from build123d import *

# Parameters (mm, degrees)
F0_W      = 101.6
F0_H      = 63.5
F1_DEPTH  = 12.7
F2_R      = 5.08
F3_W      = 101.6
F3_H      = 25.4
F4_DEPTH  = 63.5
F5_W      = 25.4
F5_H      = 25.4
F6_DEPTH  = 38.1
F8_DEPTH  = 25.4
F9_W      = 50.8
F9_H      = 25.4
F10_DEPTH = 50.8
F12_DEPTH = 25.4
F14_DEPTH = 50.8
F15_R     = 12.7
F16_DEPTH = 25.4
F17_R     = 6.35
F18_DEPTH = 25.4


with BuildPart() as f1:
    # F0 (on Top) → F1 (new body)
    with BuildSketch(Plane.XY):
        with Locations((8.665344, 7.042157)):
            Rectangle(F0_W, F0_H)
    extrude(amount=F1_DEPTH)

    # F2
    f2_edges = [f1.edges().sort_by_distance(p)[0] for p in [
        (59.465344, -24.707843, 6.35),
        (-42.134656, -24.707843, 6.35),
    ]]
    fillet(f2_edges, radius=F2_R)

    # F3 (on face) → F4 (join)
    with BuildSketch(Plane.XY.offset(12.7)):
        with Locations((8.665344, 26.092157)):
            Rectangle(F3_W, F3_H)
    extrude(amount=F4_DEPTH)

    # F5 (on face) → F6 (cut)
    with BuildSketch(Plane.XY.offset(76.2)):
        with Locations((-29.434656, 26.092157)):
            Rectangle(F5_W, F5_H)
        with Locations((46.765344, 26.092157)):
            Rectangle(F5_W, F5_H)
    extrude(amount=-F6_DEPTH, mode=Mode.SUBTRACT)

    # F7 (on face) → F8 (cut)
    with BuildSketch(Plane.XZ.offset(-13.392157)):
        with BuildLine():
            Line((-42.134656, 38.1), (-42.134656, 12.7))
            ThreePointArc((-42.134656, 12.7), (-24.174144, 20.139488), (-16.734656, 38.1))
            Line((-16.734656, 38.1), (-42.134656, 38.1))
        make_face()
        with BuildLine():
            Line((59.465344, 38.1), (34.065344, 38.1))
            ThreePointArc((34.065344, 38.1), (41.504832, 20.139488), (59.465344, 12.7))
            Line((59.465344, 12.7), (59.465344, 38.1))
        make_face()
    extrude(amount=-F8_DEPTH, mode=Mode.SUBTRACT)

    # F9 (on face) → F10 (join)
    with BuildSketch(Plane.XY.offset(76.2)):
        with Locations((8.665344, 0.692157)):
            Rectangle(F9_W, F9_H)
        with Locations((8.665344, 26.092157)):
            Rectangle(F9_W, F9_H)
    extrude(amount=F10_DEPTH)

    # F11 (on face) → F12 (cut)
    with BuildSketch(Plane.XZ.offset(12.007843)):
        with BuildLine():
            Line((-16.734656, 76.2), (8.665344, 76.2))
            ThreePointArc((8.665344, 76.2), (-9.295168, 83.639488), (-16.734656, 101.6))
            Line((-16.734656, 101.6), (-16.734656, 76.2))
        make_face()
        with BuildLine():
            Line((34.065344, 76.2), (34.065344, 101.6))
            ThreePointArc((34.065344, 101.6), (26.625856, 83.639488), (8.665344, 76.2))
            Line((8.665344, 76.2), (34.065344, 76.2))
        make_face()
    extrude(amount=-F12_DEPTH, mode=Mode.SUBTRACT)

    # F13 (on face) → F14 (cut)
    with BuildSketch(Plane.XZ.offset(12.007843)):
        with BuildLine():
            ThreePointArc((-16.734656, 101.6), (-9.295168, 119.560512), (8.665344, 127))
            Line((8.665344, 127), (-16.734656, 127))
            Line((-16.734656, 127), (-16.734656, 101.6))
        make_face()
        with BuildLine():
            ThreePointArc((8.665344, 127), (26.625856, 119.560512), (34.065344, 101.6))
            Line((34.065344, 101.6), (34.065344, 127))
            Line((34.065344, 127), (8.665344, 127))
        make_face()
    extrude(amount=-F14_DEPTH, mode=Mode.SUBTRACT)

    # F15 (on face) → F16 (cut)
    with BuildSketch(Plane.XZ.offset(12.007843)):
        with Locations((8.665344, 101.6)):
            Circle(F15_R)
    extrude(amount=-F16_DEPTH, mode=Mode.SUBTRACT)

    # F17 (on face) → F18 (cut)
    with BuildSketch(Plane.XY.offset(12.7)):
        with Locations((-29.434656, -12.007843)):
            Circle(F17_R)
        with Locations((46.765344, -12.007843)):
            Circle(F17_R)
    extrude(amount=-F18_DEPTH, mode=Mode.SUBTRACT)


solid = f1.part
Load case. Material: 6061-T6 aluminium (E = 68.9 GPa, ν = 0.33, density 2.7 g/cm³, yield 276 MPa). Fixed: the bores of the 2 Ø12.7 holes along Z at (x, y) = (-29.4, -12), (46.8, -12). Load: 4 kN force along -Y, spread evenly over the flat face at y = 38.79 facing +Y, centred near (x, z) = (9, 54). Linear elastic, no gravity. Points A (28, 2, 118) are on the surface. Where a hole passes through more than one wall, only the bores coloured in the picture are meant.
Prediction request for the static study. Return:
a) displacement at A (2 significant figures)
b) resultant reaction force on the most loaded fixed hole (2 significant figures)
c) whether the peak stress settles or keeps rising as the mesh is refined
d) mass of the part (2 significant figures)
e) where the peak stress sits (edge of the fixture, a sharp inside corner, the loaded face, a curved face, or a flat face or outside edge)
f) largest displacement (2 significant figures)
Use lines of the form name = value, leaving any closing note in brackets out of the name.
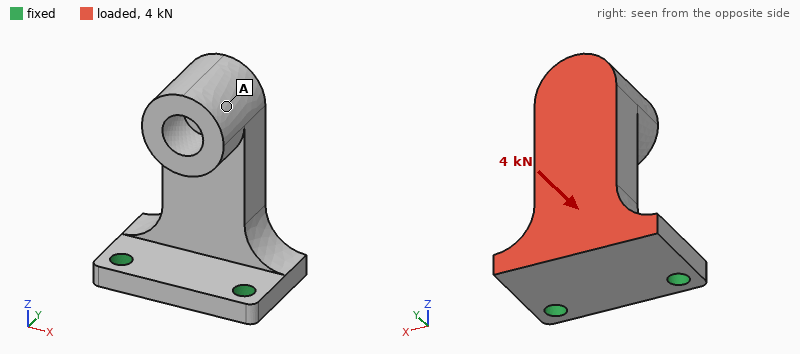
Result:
displacement at A = 0.68 mm
resultant reaction force on the most loaded fixed hole = 2.2 kN
whether the peak stress settles or keeps rising as the mesh is refined = keeps rising
mass of the part = 710 g
where the peak stress sits = edge of the fixture
largest displacement = 0.77 mm
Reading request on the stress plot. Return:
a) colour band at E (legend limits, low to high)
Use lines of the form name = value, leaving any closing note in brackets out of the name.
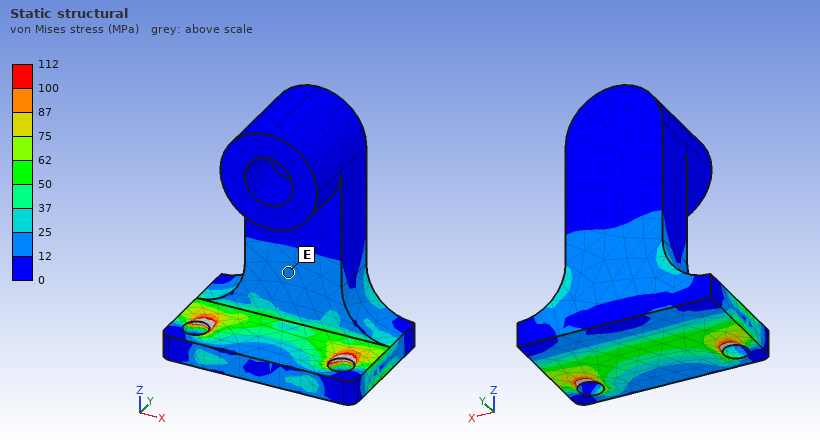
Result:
colour band at E = 12 to 25 MPa
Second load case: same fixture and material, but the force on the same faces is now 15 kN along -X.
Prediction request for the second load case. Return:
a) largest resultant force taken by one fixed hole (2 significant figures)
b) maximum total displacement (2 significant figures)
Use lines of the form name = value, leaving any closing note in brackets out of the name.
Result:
largest resultant force taken by one fixed hole = 15 kN
maximum total displacement = 0.45 mm
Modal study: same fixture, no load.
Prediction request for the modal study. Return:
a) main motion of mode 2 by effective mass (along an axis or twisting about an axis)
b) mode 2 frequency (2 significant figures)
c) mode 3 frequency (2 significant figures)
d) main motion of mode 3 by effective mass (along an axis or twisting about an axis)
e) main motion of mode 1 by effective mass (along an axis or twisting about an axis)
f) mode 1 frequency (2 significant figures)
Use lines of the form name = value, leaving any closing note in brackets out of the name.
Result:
main motion of mode 2 by effective mass = along X
mode 2 frequency = 1200 Hz
mode 3 frequency = 2400 Hz
main motion of mode 3 by effective mass = along Z
main motion of mode 1 by effective mass = along Y
mode 1 frequency = 520 Hz
